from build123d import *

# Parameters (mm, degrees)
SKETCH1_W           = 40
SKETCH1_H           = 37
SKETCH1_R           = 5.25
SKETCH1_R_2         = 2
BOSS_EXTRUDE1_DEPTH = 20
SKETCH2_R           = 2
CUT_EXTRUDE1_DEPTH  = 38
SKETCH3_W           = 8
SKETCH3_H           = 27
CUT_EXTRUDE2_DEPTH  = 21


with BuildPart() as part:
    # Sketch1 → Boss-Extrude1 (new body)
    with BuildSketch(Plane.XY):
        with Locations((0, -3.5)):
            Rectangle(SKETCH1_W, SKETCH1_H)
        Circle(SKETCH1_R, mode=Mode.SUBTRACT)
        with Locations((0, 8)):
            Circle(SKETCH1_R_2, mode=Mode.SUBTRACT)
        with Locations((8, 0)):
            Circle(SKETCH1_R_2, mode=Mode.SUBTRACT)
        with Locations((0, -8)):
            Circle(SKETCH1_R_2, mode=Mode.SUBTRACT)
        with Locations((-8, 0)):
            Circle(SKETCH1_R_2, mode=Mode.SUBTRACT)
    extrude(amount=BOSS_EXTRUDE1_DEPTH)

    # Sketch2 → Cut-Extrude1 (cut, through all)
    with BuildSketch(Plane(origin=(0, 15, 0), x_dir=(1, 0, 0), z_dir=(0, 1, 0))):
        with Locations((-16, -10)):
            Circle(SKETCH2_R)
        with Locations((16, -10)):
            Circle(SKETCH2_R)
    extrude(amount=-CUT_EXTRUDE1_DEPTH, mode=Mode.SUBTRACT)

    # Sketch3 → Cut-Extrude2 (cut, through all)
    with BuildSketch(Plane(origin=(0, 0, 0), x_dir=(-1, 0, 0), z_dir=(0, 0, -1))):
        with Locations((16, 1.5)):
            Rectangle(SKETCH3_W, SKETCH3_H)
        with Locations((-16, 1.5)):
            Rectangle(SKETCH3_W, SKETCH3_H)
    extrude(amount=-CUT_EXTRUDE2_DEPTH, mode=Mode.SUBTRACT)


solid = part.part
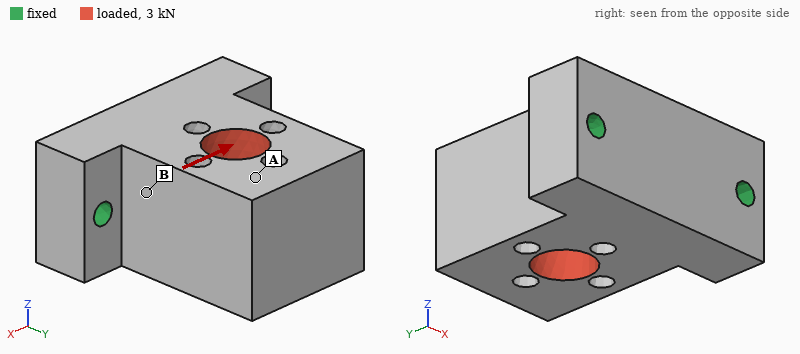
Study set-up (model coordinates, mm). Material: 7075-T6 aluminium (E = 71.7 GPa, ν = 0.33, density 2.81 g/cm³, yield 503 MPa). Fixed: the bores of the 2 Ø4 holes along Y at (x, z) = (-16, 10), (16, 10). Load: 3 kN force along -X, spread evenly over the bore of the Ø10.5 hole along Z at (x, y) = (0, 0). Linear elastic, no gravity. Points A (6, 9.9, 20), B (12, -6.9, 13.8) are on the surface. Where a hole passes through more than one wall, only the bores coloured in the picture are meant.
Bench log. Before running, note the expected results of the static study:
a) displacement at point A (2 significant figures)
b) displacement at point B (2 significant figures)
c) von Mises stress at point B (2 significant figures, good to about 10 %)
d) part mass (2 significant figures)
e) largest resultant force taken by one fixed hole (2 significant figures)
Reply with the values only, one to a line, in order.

24 µm
7.9 µm
24 MPa
51 g
2.3 kN
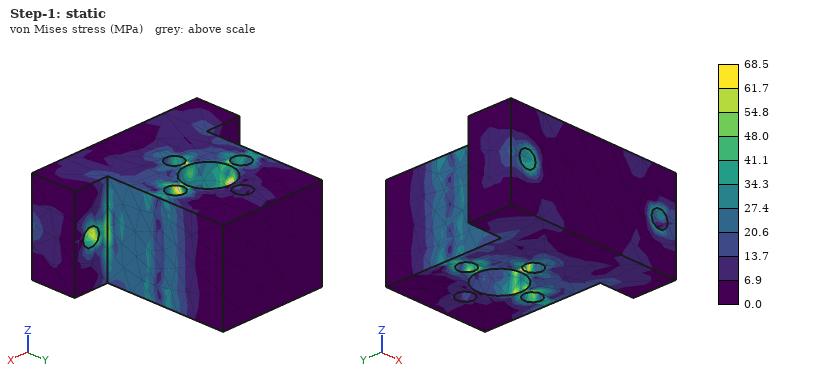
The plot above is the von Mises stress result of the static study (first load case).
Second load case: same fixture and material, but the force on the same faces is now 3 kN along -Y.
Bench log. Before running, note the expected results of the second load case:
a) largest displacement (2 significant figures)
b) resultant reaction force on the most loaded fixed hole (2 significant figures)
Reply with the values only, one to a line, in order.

7.2 µm
1.6 kN
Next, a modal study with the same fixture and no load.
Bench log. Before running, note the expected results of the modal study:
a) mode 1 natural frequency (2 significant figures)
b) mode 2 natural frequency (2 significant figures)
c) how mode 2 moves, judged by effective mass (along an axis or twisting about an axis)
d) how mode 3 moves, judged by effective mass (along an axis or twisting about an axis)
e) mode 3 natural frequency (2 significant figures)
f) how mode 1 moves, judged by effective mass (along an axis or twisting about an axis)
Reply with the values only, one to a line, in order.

6400 Hz
10 kHz
along X
twisting about Y
17 kHz
along Z
